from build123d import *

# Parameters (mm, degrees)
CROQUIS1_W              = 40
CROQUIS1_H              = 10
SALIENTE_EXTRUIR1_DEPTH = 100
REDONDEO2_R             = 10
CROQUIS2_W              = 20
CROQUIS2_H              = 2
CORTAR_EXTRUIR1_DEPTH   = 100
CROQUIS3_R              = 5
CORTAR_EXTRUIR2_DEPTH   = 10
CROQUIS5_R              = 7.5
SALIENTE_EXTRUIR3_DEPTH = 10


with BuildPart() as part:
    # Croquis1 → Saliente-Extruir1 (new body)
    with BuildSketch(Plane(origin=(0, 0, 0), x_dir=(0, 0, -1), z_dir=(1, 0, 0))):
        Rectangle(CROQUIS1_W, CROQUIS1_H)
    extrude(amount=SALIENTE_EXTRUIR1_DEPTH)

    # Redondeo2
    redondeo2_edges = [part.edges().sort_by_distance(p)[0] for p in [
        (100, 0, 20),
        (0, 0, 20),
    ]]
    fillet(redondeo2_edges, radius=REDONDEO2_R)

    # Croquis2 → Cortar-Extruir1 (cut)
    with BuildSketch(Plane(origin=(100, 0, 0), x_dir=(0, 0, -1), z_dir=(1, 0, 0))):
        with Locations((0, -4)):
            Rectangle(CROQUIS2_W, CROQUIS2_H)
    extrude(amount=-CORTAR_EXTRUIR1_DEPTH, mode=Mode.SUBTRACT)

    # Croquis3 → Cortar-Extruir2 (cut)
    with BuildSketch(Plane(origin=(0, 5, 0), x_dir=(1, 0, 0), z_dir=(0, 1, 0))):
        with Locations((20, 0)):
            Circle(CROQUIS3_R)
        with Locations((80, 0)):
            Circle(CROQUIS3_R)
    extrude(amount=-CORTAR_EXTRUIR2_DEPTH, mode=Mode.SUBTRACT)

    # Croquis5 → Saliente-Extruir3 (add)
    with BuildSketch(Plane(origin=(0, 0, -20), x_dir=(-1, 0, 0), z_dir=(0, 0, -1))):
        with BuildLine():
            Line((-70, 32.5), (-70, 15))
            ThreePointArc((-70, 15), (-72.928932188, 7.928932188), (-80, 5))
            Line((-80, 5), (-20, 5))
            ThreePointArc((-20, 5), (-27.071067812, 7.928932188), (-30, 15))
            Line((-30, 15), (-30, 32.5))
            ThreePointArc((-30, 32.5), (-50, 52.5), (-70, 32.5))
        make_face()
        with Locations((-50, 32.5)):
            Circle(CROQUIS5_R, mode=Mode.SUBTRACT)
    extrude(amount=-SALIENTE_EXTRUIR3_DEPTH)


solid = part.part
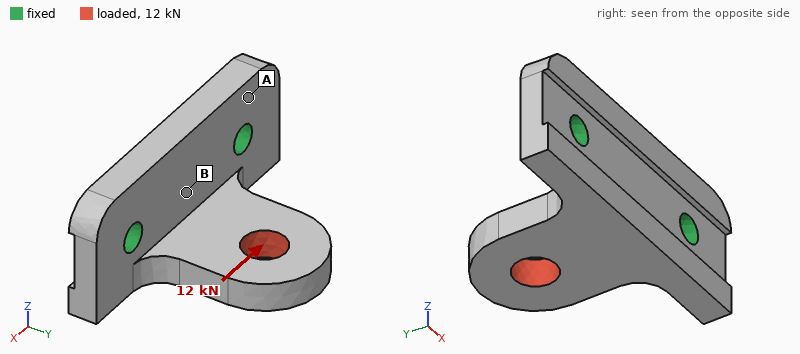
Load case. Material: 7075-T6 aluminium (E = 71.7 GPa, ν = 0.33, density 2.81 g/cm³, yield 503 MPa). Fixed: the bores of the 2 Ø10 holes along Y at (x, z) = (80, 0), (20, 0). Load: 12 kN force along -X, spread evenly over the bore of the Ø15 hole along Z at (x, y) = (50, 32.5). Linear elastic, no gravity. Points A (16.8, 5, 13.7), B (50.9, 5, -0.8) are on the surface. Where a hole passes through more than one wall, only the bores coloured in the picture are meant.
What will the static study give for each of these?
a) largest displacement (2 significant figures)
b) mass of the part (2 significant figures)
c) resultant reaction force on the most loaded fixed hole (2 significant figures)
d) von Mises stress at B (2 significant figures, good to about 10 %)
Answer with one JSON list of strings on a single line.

["0.24 mm", "140 g", "9.7 kN", "57 MPa"]
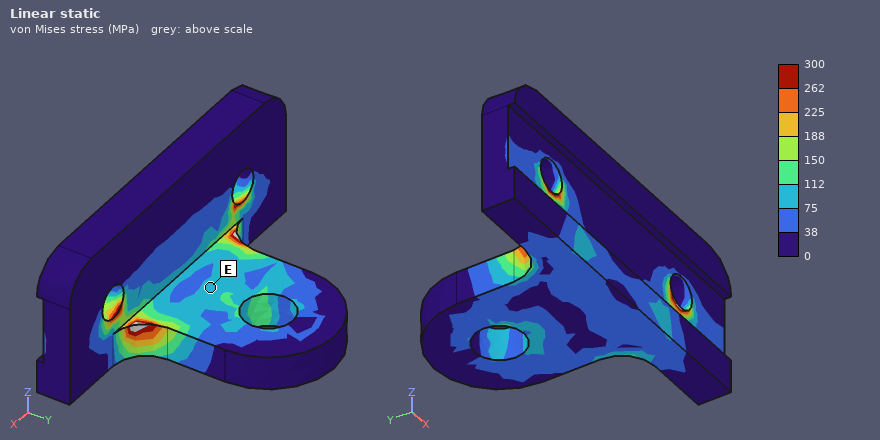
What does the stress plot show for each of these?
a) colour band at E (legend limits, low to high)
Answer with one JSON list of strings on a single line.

["75 to 112 MPa"]
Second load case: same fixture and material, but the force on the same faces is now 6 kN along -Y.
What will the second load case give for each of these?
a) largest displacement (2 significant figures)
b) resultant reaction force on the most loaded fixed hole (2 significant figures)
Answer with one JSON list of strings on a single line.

["0.16 mm", "3.1 kN"]
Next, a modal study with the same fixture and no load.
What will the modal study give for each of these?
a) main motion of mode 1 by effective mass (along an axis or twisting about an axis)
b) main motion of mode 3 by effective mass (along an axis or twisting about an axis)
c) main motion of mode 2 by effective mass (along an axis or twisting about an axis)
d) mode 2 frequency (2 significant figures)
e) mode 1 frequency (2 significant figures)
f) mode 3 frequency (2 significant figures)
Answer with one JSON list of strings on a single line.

["along Z", "along Y", "along X", "6900 Hz", "2600 Hz", "8300 Hz"]
